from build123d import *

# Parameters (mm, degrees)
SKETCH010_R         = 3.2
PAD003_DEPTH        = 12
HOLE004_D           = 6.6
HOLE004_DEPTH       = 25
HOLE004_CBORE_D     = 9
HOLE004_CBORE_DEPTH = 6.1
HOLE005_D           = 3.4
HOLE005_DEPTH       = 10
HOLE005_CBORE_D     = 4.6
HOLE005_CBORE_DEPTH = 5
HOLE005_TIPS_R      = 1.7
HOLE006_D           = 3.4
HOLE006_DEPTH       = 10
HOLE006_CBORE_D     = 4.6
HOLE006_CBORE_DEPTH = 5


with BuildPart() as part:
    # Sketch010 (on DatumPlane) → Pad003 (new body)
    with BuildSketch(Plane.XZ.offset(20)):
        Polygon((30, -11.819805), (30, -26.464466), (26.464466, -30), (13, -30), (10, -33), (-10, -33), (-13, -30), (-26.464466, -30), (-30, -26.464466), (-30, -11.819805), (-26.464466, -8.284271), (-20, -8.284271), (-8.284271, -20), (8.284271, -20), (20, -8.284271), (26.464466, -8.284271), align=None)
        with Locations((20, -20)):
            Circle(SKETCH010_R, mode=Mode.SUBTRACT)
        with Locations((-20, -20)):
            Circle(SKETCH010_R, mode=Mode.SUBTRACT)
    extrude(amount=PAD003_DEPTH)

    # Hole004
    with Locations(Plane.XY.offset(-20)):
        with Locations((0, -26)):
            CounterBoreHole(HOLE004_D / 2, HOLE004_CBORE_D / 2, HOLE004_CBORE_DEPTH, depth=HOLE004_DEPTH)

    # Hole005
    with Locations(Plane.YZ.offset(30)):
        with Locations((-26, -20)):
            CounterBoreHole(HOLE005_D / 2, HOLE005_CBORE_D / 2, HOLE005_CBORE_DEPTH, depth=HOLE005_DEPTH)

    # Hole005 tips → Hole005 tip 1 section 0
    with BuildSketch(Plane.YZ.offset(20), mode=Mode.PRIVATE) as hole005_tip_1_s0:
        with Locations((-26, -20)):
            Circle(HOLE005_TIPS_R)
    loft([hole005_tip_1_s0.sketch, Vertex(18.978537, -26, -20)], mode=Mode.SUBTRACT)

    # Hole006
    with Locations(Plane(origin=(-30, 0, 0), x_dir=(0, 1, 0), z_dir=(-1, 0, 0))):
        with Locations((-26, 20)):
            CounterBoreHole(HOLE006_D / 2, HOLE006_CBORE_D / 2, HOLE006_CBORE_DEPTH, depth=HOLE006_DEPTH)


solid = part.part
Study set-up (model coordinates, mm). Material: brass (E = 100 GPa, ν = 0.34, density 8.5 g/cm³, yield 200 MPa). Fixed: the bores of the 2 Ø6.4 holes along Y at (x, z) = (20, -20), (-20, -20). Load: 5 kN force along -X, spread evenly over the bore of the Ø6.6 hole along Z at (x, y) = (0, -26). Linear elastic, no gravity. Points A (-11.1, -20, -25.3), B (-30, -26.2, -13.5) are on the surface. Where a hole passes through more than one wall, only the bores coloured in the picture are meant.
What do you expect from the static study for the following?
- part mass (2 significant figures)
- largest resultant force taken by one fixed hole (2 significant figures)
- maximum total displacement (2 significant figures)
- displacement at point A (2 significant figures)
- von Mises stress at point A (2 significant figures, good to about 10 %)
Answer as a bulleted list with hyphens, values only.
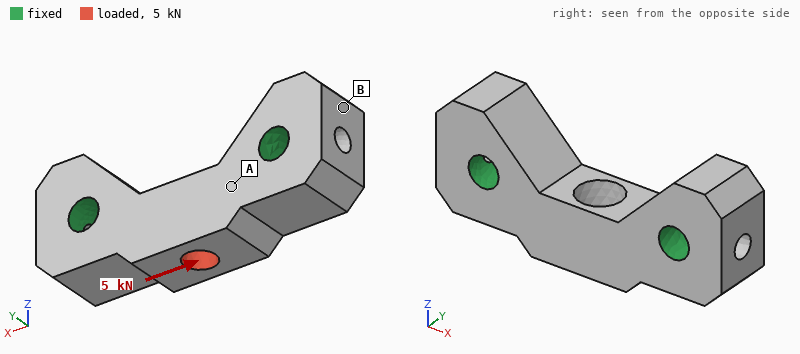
- 90 g
- 2.7 kN
- 6.1 µm
- 2.1 µm
- 19 MPa
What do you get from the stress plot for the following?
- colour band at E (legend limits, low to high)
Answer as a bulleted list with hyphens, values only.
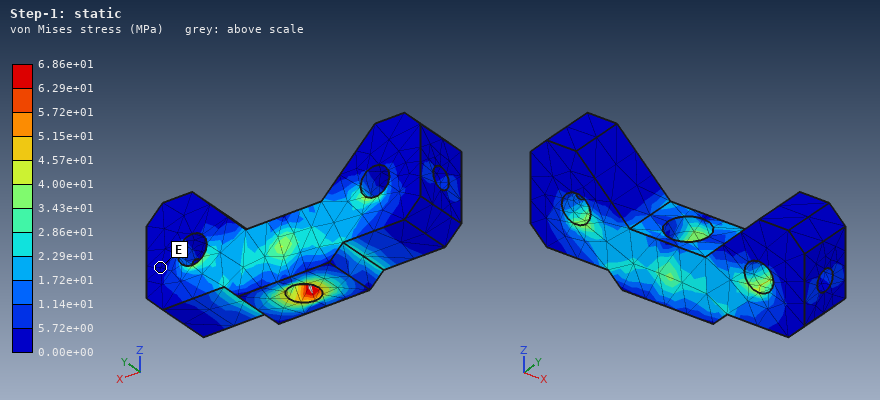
- 0.00e+00 to 5.72e+00 MPa
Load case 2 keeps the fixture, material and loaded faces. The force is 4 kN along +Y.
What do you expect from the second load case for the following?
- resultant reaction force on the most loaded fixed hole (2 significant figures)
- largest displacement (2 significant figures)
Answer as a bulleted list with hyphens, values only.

- 2.0 kN
- 27 µm
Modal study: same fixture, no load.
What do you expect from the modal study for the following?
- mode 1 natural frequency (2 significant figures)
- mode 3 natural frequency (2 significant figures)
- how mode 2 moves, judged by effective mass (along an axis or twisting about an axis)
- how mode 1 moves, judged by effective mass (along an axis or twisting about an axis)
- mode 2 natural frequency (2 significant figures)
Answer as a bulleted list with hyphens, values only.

- 18 kHz
- 28 kHz
- along Z
- along Y
- 22 kHz
